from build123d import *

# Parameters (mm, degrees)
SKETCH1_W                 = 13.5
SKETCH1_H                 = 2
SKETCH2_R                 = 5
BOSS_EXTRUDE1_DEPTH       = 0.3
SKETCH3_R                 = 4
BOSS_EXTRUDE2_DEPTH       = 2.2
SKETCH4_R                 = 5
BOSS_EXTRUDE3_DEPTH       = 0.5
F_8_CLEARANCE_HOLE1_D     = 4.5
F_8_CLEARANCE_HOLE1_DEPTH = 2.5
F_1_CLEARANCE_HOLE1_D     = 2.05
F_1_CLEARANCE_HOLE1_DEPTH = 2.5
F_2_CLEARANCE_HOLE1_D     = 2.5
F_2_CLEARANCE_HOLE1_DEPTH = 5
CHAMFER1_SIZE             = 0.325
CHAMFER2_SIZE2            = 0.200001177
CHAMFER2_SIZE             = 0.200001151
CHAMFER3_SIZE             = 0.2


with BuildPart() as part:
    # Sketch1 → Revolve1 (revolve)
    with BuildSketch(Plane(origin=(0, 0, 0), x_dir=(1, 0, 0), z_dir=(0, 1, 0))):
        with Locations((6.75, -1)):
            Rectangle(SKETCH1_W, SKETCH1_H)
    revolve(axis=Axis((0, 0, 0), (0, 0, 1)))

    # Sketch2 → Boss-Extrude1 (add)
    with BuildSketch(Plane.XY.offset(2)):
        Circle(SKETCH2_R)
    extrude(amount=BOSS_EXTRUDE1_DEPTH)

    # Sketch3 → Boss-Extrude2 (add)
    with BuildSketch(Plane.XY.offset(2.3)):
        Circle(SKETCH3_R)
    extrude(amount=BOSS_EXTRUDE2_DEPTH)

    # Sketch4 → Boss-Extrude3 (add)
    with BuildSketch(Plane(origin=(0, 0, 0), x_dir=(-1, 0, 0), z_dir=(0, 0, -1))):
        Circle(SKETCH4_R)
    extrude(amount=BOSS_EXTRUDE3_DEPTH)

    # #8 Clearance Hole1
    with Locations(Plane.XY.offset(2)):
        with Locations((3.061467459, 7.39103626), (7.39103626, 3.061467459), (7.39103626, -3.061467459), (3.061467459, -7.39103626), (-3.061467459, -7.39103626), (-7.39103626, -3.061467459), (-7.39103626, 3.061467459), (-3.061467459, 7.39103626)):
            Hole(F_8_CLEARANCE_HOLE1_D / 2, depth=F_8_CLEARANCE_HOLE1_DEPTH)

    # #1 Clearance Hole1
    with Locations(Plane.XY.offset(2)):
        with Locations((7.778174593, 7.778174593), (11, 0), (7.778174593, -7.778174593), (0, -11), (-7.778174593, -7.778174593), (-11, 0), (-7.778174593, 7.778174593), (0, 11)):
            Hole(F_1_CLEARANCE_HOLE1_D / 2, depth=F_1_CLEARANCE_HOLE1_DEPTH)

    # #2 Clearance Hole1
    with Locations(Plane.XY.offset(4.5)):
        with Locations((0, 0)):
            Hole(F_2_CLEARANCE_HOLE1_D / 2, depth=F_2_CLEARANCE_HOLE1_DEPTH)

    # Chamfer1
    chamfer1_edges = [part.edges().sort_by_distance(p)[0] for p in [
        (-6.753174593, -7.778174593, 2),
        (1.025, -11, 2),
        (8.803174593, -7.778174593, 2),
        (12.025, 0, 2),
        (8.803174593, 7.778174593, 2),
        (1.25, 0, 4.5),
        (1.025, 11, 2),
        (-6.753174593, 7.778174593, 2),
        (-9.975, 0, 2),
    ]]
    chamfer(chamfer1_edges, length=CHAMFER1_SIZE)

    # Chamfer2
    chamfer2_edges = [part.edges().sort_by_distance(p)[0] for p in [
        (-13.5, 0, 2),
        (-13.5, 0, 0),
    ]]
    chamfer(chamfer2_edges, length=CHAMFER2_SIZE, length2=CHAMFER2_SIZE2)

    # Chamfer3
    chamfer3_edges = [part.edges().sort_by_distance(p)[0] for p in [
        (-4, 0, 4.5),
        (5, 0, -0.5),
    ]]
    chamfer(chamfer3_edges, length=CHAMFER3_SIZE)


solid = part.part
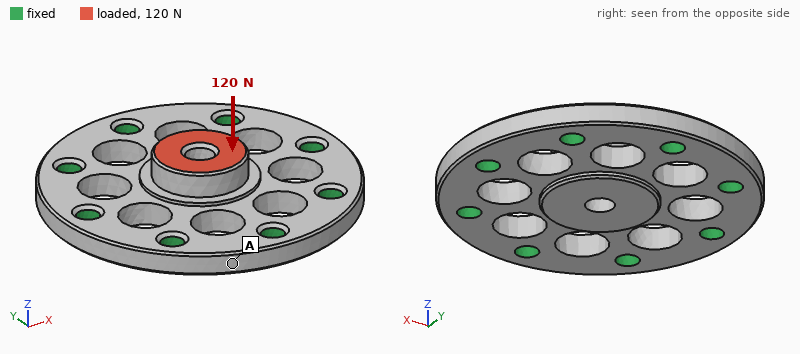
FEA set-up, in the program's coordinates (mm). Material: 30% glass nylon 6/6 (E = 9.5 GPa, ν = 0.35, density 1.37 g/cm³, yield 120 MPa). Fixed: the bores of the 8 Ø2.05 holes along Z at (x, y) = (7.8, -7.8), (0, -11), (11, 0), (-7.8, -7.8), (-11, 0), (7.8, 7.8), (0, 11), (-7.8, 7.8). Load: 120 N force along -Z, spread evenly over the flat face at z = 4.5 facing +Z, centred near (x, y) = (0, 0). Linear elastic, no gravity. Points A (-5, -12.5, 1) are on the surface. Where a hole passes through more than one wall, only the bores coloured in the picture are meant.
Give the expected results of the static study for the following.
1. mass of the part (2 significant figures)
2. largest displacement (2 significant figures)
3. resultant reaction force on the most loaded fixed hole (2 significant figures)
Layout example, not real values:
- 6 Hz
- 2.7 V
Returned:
- 1.3 g
- 25 µm
- 16 N
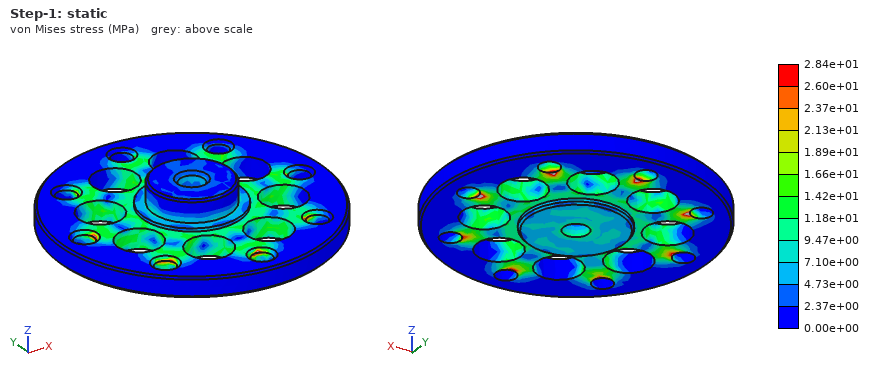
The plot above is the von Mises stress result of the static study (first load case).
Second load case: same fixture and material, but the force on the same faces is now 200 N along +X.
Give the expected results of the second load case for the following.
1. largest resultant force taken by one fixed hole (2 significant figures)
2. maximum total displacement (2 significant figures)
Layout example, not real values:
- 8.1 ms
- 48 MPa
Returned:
- 49 N
- 31 µm
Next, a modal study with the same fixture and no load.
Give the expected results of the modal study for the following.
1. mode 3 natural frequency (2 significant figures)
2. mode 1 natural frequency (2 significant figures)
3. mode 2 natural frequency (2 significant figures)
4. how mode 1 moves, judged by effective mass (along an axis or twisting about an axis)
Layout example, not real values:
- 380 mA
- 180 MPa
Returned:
- 28 kHz
- 16 kHz
- 28 kHz
- along Z
